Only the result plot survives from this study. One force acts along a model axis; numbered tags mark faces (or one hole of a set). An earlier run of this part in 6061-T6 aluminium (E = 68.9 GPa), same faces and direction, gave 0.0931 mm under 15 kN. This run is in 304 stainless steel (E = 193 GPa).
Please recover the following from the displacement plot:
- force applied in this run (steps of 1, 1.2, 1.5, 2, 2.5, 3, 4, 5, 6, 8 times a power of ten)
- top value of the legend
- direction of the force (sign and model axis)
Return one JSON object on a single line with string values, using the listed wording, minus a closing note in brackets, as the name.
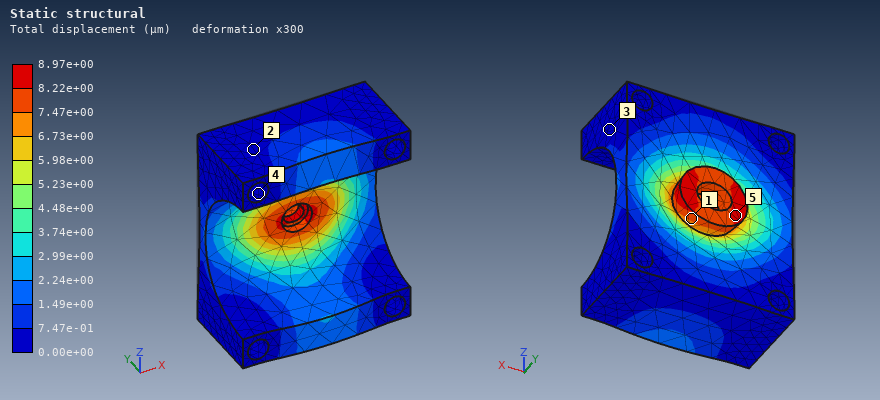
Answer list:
{"force applied in this run": "4 kN", "top value of the legend": "8.97e+00 µm", "direction of the force": "-Y"}
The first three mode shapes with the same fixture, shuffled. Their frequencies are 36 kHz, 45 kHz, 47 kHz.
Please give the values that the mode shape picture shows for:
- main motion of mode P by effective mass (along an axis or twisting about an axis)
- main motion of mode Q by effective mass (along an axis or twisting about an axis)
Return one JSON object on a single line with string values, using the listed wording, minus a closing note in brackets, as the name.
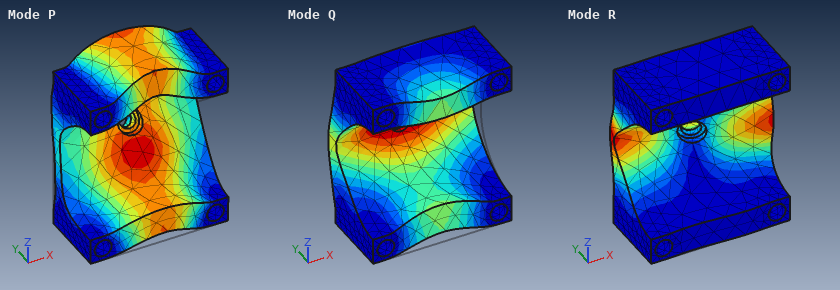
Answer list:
{"main motion of mode P by effective mass": "along Z", "main motion of mode Q by effective mass": "along Y"}
